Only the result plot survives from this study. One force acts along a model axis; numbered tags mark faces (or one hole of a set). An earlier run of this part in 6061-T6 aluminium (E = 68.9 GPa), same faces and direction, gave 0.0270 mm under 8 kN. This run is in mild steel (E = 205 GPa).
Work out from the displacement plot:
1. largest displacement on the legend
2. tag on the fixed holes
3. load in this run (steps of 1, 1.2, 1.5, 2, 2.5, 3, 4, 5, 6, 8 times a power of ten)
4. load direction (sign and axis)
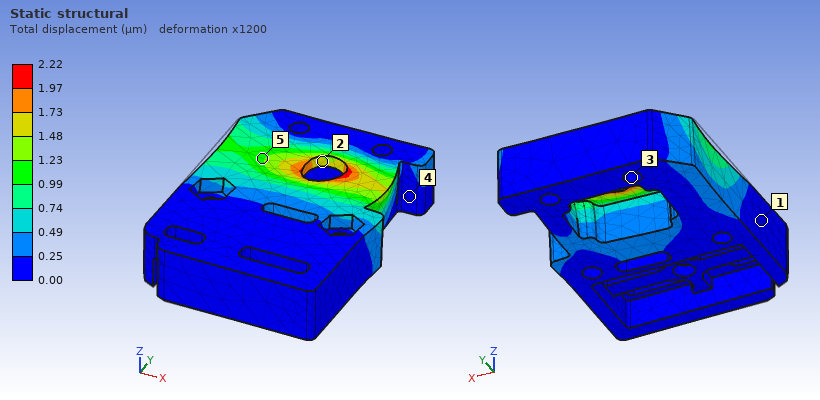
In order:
2.22 µm
3
2 kN
+X
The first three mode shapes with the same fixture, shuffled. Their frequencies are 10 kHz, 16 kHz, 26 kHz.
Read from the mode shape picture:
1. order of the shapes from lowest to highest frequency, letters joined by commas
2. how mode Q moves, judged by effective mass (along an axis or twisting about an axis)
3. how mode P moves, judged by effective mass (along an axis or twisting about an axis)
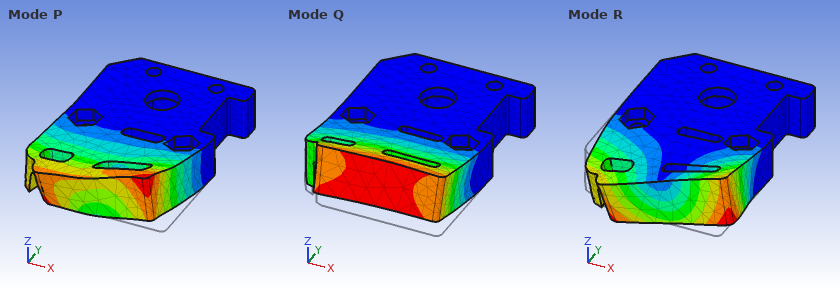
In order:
Q, R, P
along Z
along X
